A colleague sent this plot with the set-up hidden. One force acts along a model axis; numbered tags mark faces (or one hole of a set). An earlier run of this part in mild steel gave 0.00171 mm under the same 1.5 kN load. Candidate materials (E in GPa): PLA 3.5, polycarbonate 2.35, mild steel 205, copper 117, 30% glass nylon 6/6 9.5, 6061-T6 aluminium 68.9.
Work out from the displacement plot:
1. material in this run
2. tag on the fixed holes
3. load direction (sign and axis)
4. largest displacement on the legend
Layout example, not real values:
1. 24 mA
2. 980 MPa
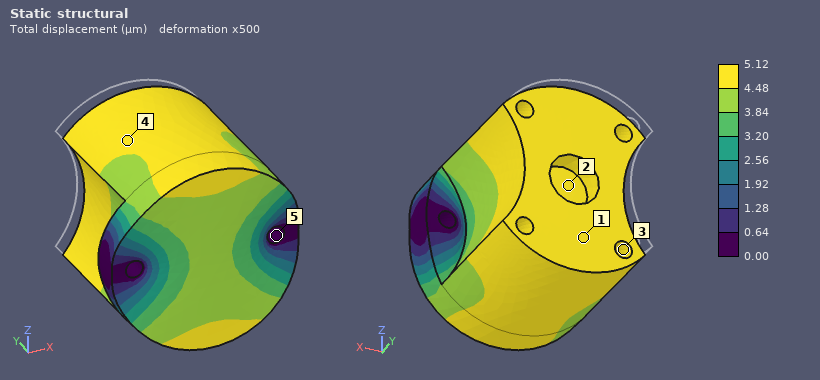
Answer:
1. 6061-T6 aluminium
2. 5
3. -Y
4. 5.12 µm
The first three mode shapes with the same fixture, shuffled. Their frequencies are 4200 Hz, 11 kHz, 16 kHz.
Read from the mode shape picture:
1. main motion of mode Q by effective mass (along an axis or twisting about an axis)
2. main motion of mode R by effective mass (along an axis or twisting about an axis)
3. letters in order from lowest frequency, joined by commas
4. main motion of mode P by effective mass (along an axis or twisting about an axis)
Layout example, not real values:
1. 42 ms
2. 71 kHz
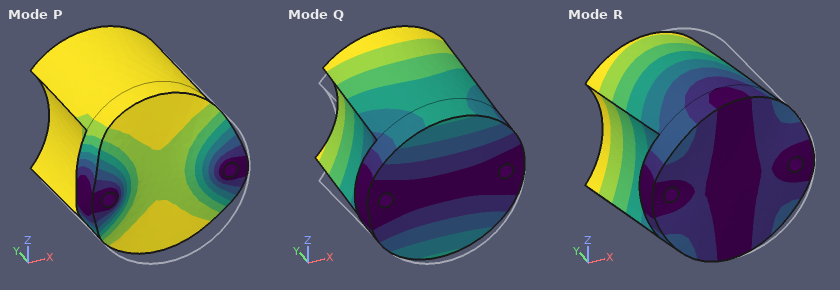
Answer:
1. along Z
2. along X
3. Q, R, P
4. along Y
